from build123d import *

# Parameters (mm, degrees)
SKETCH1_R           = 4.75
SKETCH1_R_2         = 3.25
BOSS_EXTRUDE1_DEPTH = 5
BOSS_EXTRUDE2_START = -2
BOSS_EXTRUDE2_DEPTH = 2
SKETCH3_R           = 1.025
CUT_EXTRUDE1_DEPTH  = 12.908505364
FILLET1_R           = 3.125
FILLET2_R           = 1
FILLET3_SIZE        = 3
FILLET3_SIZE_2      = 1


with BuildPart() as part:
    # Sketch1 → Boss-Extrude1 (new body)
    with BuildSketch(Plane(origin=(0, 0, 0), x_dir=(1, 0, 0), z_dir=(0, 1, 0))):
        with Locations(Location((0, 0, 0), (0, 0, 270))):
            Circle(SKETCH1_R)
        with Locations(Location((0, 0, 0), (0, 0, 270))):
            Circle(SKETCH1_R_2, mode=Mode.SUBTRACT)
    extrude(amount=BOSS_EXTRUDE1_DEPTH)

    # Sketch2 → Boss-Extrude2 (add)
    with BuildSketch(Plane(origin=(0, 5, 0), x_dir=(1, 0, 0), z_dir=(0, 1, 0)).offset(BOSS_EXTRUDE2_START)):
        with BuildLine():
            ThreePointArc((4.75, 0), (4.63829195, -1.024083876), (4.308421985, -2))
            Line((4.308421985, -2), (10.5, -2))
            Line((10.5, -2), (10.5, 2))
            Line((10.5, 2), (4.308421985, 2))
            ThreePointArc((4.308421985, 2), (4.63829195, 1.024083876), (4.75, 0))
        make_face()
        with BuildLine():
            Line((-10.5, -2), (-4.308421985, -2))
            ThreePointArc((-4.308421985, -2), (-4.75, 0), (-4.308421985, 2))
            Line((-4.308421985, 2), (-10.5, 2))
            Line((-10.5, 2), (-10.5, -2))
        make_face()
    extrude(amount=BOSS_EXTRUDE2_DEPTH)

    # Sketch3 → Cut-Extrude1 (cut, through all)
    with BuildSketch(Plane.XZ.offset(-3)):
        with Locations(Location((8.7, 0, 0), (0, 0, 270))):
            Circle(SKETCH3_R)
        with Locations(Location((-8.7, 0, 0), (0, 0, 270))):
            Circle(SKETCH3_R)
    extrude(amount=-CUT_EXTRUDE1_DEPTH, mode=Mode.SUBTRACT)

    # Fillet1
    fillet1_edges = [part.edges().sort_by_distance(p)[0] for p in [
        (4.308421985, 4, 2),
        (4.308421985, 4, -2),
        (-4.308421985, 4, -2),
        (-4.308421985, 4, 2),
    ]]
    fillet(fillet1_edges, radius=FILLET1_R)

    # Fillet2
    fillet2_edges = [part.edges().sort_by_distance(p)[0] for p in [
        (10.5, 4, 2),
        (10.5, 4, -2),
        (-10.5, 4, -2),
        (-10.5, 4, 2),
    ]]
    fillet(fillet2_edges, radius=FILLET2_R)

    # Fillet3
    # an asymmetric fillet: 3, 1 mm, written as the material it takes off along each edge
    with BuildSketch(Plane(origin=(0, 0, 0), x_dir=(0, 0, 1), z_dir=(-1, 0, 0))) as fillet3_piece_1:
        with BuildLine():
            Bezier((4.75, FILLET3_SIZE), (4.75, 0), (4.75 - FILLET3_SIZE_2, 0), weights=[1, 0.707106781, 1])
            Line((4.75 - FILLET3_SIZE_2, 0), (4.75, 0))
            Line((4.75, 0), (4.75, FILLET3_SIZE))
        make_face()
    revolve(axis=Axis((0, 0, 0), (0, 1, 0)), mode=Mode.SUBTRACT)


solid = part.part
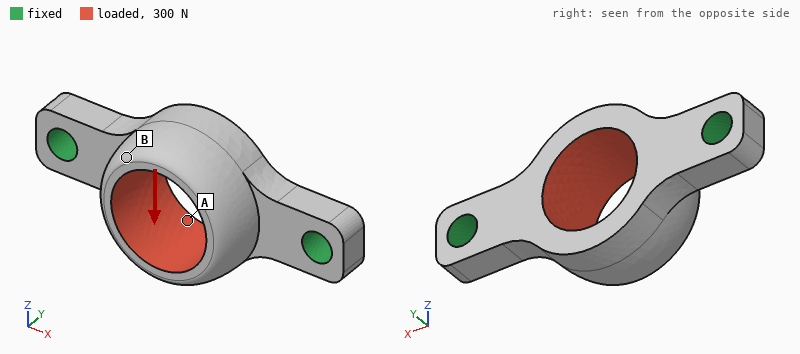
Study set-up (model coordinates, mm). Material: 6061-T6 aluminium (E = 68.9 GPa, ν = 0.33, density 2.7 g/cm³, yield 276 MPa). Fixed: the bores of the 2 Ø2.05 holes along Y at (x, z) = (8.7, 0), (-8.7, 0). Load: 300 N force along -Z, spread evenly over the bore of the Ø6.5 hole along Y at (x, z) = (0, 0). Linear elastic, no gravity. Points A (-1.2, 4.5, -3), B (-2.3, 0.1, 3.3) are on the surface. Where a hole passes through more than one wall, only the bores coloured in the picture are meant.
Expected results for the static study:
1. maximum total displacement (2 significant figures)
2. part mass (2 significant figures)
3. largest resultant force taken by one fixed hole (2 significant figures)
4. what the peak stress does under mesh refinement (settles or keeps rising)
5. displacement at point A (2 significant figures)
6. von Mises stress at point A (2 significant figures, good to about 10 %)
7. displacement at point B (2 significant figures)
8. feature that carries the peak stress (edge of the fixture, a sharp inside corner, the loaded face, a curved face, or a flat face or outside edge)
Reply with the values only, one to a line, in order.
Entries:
30 µm
0.68 g
150 N
keeps rising
14 µm
33 MPa
28 µm
edge of the fixture
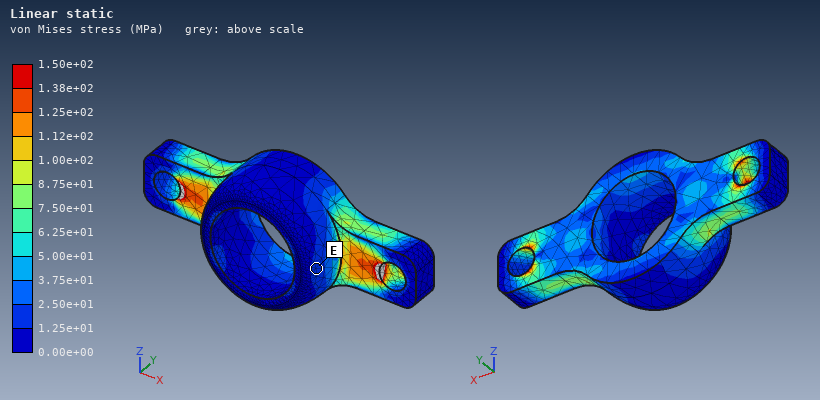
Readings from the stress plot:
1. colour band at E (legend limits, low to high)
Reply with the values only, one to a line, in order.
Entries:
1.25e+01 to 2.50e+01 MPa
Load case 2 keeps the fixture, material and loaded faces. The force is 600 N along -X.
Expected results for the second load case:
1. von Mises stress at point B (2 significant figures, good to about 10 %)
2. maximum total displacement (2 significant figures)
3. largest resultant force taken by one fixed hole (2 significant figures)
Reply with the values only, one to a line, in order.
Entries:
21 MPa
7.3 µm
310 N
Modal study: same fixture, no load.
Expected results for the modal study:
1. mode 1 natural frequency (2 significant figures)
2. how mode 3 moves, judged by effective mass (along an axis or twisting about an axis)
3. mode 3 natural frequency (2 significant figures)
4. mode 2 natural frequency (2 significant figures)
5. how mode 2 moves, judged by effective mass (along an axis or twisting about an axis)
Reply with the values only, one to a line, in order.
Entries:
22 kHz
along Z
54 kHz
31 kHz
along Y
